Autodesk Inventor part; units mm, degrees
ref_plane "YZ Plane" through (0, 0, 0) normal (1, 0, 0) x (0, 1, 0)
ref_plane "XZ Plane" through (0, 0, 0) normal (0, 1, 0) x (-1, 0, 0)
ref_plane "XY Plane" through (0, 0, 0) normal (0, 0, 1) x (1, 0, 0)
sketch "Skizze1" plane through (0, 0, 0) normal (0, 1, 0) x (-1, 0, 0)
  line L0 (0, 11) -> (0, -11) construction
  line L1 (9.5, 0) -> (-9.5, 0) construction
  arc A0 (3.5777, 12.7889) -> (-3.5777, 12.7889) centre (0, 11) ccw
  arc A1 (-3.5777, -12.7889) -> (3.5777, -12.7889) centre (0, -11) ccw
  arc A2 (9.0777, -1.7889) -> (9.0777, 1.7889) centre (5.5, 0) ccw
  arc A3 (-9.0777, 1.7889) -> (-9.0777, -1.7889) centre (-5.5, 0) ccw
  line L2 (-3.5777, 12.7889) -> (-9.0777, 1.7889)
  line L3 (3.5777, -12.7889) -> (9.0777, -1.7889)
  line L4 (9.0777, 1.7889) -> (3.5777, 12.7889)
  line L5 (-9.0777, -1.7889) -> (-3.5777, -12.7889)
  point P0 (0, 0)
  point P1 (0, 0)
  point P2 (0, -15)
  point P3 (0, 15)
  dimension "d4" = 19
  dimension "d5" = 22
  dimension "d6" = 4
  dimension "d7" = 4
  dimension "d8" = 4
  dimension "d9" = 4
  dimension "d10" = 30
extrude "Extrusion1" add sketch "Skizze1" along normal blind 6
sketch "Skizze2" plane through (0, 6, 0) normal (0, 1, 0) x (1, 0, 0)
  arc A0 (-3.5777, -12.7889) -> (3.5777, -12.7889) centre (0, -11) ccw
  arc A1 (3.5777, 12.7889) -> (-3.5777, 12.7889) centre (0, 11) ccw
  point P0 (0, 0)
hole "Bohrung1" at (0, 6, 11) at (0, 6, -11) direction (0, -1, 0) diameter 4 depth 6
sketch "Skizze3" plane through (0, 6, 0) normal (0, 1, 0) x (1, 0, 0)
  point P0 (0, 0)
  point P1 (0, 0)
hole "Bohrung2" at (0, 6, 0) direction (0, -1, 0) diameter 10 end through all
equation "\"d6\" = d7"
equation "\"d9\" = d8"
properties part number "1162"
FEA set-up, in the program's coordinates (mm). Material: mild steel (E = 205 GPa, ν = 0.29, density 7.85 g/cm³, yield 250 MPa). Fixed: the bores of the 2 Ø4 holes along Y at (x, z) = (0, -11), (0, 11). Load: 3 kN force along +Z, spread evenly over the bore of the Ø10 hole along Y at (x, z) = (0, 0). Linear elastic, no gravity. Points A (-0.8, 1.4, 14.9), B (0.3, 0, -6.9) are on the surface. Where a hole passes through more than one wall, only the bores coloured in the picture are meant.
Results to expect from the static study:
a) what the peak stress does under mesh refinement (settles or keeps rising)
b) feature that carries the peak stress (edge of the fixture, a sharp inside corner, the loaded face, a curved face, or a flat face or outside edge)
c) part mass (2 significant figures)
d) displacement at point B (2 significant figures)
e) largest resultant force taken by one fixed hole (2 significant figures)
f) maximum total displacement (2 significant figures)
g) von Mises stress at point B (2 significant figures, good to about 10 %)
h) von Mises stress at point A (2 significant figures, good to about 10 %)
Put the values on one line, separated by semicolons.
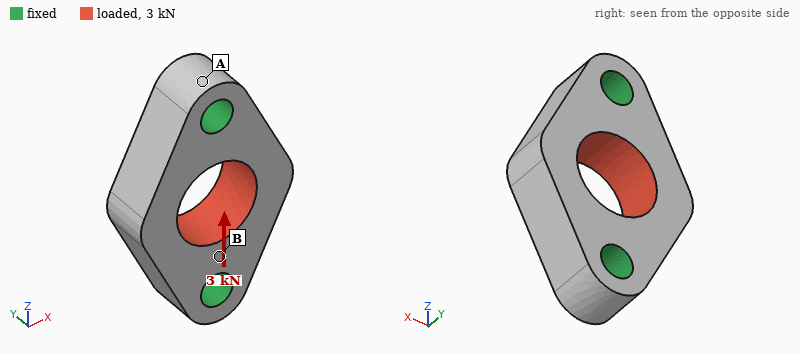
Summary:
keeps rising; edge of the fixture; 12 g; 0.29 µm; 1.5 kN; 1.5 µm; 25 MPa; 6.9 MPa
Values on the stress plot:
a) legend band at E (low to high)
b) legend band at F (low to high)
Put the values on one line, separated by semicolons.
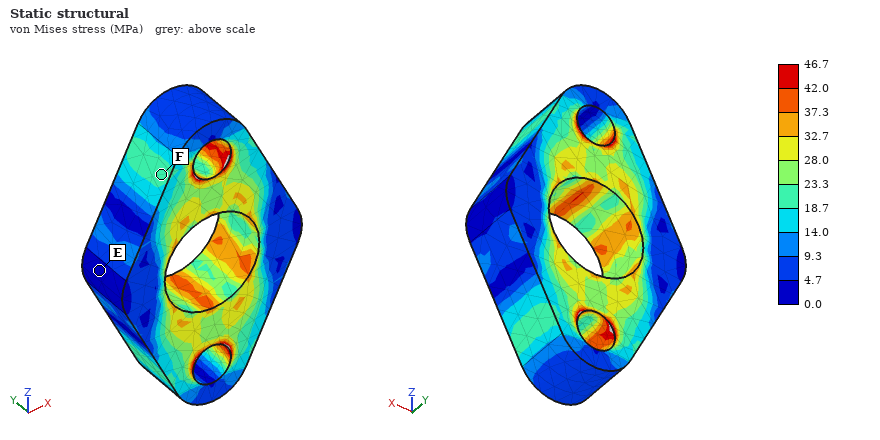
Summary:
0.0 to 4.7 MPa; 18.7 to 23.3 MPa
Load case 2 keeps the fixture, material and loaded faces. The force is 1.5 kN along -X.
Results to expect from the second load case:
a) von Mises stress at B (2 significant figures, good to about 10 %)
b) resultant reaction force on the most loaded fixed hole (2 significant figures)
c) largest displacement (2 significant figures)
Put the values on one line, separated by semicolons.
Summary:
22 MPa; 750 N; 1.4 µm
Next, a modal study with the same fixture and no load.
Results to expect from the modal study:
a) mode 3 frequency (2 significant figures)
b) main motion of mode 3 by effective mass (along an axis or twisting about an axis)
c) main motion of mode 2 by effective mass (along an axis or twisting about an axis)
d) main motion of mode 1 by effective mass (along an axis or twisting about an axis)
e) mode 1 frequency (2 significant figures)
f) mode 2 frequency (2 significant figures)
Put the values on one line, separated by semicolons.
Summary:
70 kHz; along X; along Y; twisting about Z; 38 kHz; 42 kHz
